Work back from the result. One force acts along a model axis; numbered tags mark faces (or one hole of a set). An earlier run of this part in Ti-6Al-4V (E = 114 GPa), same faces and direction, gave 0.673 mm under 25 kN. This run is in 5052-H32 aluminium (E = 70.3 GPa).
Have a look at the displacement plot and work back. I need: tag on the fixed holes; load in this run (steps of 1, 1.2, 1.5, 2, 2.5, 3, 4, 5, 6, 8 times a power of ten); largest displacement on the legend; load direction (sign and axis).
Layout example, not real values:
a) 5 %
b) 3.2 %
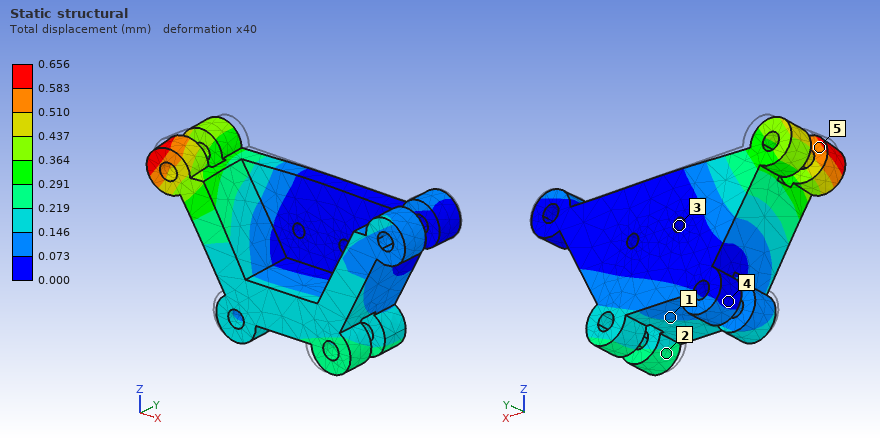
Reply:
a) 3
b) 15 kN
c) 0.656 mm
d) -Y
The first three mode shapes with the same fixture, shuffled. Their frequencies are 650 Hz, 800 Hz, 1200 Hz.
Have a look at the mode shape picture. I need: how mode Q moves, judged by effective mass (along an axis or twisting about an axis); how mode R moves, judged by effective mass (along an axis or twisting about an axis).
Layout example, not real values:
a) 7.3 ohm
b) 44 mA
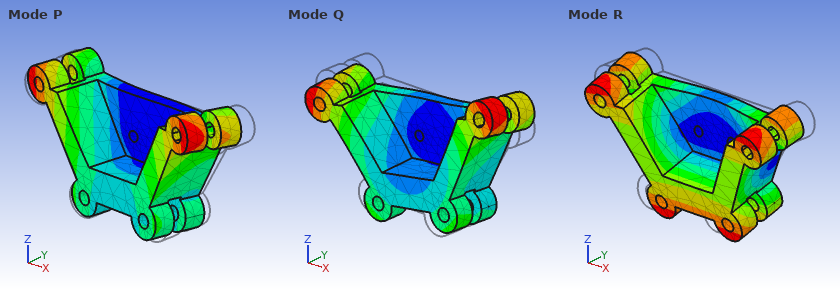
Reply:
a) twisting about Y
b) along Z
